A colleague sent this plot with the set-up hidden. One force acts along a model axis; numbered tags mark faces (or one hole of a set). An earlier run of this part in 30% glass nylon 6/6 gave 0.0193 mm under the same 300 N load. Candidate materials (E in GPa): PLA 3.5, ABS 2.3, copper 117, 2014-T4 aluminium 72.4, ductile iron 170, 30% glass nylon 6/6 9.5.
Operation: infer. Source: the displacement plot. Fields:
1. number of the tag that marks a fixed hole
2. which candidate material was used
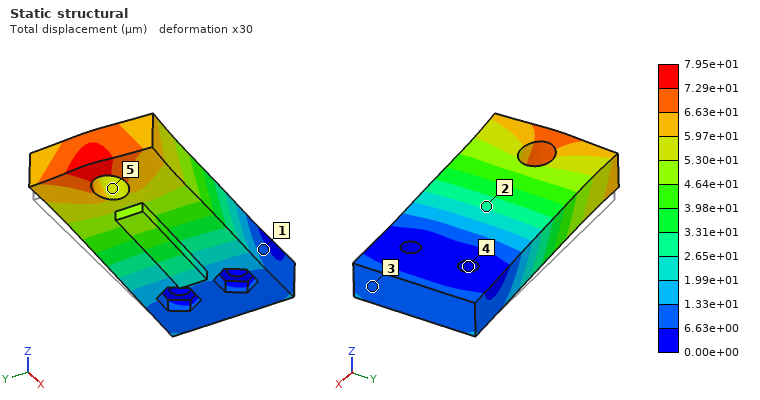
4
ABS
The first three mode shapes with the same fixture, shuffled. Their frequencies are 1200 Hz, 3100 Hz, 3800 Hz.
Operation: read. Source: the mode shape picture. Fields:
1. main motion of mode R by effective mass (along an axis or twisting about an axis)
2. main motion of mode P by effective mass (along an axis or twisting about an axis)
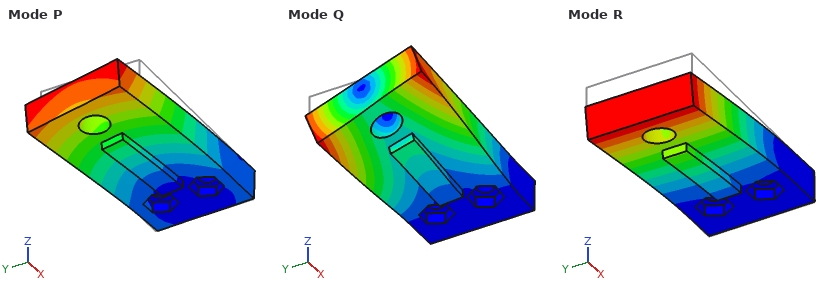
along Z
along Y
